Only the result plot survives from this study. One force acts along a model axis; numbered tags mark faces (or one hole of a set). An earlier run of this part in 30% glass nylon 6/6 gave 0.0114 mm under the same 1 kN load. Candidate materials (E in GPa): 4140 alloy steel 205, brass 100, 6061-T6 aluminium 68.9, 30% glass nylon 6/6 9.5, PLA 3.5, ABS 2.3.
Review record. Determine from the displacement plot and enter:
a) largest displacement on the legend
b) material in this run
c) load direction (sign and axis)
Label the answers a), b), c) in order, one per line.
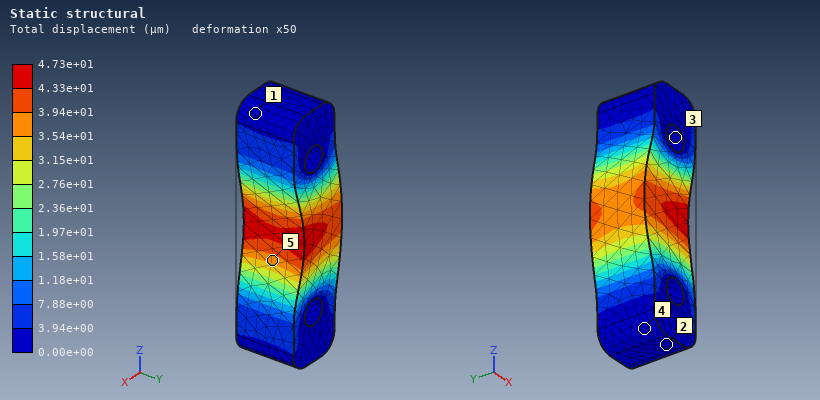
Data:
a) 4.73e+01 µm
b) ABS
c) -X
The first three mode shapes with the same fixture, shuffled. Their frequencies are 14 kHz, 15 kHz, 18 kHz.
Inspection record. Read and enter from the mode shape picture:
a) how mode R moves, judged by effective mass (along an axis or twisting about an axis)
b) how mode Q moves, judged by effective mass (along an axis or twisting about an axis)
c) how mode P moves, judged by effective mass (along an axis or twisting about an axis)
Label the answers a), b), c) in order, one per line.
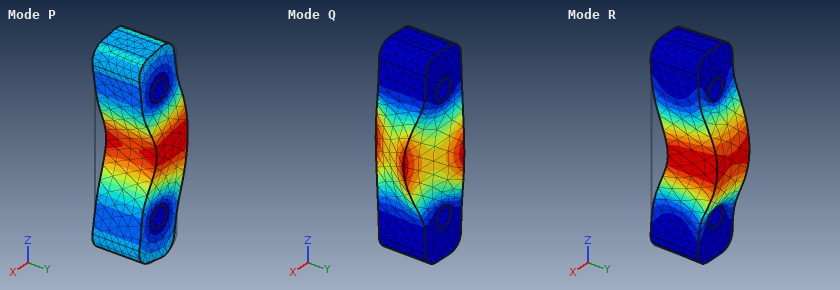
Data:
a) along Y
b) twisting about Z
c) along X
